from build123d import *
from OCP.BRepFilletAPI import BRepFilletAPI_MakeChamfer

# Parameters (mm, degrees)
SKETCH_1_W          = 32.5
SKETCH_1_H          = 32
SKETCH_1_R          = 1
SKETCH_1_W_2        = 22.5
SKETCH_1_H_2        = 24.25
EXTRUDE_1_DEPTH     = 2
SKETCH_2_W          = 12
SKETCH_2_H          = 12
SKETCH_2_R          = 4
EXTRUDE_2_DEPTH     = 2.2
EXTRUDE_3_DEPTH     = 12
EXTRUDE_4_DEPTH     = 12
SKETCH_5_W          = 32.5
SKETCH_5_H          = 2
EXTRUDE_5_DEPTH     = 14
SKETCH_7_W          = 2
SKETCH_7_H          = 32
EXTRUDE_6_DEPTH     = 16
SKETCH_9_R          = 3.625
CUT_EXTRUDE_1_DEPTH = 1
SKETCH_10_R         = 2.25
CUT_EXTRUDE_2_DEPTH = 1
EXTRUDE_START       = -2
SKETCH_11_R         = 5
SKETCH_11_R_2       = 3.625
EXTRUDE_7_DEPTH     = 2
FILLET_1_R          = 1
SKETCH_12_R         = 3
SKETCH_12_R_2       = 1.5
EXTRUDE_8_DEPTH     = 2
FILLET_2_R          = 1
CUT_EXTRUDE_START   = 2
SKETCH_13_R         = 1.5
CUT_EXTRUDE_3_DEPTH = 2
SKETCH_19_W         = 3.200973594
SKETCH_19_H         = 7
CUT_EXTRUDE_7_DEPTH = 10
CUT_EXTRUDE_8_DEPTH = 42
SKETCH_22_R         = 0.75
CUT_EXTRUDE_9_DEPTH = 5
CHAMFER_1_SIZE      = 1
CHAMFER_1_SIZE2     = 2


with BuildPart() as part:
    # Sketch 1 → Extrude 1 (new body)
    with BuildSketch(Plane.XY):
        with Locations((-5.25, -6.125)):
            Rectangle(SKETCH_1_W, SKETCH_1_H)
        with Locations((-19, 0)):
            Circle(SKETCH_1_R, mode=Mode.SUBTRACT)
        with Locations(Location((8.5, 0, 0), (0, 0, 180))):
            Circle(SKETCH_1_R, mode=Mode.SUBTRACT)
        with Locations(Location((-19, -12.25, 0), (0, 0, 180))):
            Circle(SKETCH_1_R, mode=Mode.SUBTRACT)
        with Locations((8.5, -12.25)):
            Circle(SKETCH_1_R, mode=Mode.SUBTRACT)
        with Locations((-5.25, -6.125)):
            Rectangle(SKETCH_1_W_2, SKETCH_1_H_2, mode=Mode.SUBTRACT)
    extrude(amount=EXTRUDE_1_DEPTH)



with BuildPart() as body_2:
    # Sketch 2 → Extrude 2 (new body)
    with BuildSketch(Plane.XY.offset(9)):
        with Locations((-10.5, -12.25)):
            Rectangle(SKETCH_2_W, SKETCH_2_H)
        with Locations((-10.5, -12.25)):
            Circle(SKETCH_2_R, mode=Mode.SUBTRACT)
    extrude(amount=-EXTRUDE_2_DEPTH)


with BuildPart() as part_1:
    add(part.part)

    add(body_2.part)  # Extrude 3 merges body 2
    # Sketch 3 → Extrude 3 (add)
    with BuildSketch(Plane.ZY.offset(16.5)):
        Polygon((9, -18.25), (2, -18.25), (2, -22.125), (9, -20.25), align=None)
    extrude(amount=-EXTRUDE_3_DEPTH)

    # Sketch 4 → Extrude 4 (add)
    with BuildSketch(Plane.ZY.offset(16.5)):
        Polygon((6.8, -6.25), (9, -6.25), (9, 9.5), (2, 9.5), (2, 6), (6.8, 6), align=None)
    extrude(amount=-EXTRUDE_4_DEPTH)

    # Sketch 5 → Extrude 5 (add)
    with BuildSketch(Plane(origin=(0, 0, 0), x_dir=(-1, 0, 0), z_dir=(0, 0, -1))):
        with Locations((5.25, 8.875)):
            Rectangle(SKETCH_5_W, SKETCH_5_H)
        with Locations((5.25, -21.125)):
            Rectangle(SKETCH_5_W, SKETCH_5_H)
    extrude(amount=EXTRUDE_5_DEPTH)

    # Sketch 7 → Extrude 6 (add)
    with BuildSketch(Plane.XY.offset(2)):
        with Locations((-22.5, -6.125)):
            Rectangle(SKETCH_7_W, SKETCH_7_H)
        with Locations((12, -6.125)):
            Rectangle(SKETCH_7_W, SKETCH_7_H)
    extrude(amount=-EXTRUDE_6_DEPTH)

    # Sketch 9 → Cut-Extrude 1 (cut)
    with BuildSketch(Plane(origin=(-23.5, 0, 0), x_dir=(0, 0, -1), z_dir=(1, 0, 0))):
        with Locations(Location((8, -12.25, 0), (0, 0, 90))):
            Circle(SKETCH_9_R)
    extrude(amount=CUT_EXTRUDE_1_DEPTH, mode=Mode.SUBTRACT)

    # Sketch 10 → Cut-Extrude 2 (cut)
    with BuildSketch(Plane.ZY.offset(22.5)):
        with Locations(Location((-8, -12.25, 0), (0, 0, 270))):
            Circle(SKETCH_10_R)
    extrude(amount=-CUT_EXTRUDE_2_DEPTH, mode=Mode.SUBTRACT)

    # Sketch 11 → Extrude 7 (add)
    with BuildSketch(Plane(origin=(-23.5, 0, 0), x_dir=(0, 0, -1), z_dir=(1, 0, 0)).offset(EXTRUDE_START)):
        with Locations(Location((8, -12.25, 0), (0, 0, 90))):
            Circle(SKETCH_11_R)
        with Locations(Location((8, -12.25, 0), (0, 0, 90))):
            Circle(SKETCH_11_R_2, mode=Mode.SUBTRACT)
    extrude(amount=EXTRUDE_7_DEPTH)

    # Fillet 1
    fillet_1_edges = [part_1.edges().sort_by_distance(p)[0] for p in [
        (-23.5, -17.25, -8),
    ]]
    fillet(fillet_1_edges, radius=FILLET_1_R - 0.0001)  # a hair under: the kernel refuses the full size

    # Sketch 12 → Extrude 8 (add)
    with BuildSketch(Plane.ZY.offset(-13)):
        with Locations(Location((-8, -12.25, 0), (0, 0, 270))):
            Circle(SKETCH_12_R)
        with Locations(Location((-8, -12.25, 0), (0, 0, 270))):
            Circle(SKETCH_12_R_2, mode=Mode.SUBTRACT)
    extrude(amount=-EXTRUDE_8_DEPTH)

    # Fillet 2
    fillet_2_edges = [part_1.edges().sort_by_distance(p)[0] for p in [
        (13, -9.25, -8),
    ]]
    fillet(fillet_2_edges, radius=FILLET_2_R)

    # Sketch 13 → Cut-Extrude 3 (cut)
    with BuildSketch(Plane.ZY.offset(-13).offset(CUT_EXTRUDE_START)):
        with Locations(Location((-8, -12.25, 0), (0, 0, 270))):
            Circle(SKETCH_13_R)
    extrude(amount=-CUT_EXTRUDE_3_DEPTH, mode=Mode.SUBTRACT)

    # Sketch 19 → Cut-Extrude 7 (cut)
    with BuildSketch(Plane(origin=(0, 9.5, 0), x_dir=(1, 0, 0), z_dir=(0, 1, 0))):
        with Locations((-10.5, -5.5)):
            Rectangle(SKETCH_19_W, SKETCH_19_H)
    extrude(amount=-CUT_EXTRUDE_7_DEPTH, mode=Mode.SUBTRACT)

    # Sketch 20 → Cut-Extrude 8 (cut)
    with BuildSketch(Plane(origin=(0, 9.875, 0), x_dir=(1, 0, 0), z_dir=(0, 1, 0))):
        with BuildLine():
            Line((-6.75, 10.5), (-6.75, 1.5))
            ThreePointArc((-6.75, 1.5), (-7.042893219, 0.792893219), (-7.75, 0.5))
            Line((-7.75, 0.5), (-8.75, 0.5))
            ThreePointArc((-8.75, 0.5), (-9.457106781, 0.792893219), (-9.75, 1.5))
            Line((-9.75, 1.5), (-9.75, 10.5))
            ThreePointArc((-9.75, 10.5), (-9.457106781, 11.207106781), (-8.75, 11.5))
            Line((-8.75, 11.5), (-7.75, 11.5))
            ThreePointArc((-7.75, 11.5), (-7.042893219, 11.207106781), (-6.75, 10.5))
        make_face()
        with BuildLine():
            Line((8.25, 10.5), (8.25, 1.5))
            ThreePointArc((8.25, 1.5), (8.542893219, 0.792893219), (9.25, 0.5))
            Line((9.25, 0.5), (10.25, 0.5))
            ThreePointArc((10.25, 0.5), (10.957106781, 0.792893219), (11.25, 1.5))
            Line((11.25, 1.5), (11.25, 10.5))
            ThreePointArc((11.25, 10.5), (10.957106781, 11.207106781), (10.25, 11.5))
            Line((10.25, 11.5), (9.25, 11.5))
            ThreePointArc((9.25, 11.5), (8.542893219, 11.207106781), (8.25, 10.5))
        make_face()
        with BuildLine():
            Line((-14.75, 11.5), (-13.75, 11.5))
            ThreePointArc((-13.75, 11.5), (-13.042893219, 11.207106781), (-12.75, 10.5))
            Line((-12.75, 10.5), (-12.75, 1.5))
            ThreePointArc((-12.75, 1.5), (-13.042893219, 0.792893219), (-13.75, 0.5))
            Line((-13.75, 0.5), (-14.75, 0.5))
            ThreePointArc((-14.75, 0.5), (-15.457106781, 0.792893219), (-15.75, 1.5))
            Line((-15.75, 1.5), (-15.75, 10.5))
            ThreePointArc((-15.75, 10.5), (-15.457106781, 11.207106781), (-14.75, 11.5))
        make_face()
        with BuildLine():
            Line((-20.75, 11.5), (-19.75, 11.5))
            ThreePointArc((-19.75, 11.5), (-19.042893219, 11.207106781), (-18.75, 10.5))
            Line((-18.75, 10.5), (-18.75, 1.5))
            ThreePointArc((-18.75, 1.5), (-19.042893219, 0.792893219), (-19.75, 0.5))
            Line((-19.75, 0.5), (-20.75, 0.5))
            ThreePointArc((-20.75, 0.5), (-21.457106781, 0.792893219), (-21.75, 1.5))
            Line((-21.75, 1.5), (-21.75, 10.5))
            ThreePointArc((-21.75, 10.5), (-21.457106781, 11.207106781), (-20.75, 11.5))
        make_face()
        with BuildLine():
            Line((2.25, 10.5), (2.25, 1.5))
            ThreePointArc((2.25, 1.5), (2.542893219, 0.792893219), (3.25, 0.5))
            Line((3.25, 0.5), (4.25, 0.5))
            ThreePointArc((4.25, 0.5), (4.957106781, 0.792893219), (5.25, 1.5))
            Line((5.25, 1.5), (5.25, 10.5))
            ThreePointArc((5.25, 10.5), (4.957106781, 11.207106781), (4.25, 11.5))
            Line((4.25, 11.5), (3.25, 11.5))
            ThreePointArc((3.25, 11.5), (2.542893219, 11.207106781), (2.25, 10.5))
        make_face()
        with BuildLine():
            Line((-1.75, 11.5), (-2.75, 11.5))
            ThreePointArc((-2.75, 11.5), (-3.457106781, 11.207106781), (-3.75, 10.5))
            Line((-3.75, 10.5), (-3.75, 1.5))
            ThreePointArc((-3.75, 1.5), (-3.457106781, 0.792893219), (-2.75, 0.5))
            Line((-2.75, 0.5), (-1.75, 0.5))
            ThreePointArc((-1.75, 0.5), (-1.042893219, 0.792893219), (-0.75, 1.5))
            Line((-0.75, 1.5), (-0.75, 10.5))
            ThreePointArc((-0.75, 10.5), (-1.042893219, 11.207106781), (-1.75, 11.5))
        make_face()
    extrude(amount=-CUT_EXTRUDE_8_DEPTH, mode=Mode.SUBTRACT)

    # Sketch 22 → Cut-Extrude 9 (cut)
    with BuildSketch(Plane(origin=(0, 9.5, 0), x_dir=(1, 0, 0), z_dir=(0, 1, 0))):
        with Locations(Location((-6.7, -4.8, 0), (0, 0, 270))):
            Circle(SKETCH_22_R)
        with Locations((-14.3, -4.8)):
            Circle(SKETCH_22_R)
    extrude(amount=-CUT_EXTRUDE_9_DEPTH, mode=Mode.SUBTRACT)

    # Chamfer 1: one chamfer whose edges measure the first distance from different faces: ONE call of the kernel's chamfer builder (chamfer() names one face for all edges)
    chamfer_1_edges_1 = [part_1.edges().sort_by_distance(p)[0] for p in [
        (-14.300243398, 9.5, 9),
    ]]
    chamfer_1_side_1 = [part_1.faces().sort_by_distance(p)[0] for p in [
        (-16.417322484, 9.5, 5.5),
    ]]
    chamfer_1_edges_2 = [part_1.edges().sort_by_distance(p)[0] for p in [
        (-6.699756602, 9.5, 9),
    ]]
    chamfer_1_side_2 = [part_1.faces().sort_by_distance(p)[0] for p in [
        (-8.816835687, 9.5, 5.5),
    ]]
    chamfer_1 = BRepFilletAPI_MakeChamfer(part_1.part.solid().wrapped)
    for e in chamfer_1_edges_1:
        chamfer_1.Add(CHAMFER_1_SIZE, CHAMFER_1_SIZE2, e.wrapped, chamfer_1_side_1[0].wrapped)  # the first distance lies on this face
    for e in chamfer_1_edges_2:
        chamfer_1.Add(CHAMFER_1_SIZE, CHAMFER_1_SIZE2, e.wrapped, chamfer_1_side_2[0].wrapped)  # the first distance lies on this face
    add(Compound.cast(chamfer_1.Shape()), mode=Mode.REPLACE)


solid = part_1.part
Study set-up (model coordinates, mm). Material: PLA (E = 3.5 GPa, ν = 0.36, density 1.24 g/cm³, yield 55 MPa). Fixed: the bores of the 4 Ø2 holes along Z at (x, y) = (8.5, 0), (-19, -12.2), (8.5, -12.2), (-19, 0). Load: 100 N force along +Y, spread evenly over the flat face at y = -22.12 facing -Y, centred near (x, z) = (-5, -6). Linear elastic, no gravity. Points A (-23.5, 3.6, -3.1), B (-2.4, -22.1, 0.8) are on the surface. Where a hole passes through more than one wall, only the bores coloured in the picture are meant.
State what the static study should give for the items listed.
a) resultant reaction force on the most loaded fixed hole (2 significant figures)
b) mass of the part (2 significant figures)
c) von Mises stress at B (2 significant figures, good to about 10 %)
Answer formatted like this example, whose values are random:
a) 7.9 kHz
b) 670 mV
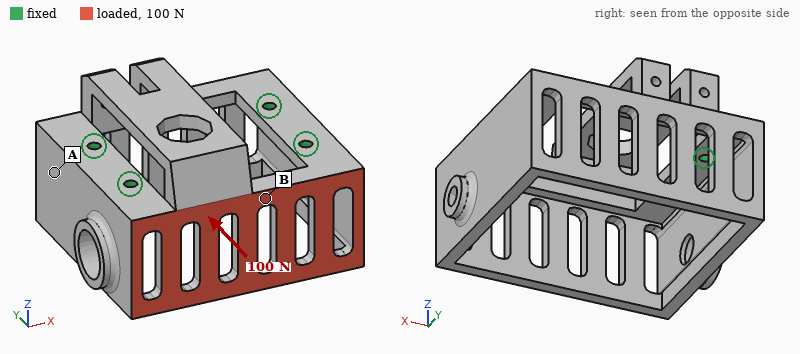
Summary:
a) 58 N
b) 6.1 g
c) 11 MPa
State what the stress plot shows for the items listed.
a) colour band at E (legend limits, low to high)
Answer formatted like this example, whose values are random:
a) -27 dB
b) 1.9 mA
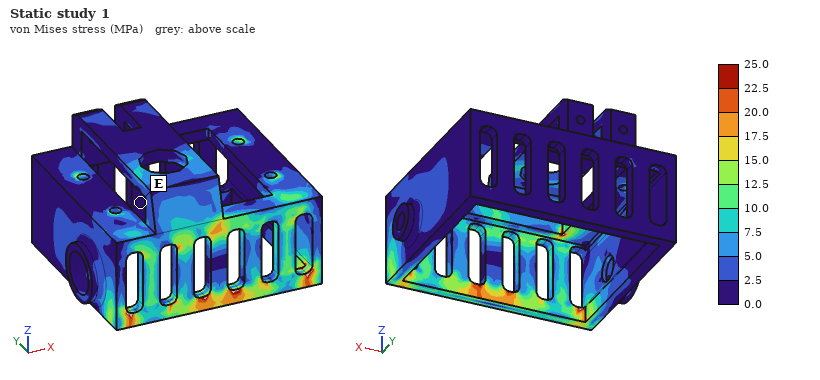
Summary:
a) 0.0 to 2.5 MPa
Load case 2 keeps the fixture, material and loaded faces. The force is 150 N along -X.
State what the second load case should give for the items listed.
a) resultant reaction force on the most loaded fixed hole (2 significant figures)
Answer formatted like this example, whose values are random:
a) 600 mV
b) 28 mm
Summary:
a) 100 N
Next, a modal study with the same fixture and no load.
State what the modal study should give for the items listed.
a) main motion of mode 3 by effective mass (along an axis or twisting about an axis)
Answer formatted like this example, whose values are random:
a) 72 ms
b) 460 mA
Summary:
a) along X
